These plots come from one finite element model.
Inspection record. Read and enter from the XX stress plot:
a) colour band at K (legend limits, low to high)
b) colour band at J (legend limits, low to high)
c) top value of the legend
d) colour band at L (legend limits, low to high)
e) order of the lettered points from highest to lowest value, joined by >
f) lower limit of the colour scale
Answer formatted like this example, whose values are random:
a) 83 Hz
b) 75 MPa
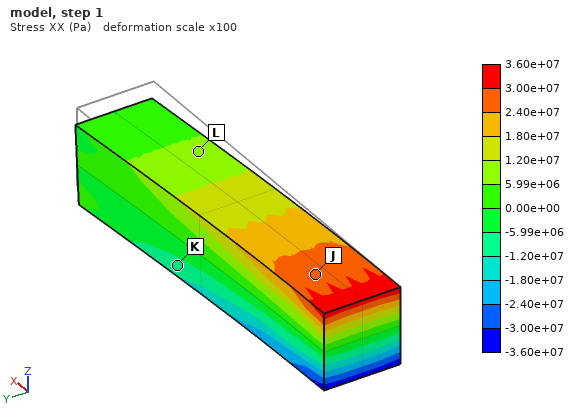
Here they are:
a) -1.20e+07 to -5.99e+06 Pa
b) 2.40e+07 to 3.00e+07 Pa
c) 3.60e+07 Pa
d) 5.99e+06 to 1.20e+07 Pa
e) J > L > K
f) -3.60e+07 Pa
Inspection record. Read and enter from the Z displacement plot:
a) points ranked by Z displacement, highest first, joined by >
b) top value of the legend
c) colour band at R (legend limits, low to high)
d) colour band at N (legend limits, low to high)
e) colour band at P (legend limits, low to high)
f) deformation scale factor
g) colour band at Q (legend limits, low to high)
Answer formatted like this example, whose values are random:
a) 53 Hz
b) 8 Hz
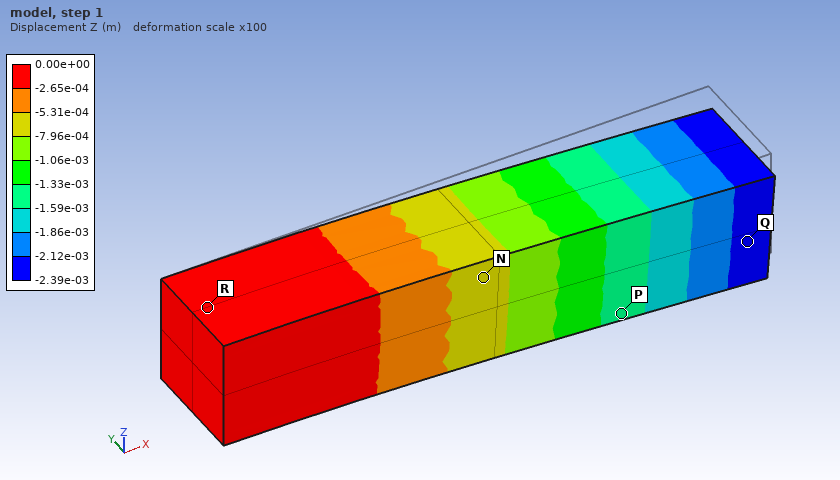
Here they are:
a) R > N > P > Q
b) 0.00e+00 m
c) -2.65e-04 to 0.00e+00 m
d) -7.96e-04 to -5.31e-04 m
e) -1.59e-03 to -1.33e-03 m
f) 100
g) -2.39e-03 to -2.12e-03 m
